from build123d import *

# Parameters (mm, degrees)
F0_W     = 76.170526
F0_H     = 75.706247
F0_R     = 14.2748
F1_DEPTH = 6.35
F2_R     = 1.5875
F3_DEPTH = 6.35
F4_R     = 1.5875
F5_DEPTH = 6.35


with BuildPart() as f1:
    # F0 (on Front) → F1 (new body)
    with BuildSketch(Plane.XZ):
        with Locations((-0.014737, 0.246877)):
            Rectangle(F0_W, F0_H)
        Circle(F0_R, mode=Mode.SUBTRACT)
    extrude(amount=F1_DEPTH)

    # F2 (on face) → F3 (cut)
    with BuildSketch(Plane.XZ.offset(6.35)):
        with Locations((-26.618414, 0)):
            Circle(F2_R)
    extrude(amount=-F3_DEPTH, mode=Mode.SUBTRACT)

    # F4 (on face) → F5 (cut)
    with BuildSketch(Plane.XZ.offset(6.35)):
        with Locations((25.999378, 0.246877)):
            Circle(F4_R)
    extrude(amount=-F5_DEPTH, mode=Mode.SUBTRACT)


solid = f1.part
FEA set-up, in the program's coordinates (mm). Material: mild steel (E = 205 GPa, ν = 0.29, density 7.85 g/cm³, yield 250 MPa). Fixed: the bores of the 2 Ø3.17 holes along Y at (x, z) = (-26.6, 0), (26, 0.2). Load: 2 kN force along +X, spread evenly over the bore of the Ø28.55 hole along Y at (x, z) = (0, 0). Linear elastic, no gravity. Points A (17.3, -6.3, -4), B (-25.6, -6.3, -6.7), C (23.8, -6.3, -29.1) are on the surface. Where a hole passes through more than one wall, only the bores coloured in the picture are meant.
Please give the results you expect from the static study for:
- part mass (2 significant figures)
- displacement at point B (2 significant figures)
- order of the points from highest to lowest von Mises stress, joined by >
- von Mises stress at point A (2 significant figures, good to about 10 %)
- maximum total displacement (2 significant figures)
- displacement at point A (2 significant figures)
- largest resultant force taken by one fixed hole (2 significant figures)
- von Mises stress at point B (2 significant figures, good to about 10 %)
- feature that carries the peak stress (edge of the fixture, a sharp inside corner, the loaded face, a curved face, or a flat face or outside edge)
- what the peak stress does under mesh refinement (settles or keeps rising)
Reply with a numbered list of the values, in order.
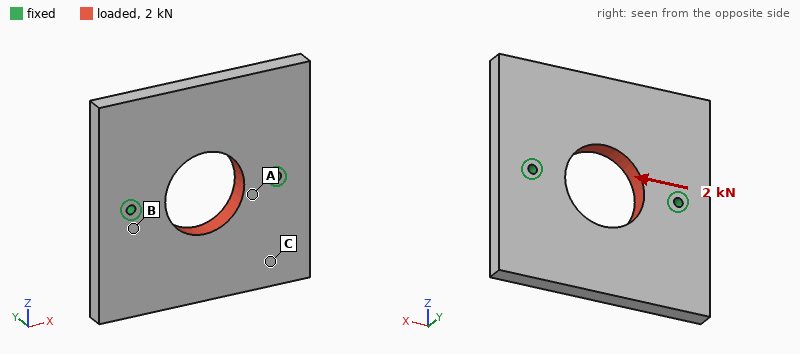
1. 250 g
2. 0.42 µm
3. A > B > C
4. 7.5 MPa
5. 1.1 µm
6. 0.47 µm
7. 1.0 kN
8. 4.5 MPa
9. edge of the fixture
10. keeps rising
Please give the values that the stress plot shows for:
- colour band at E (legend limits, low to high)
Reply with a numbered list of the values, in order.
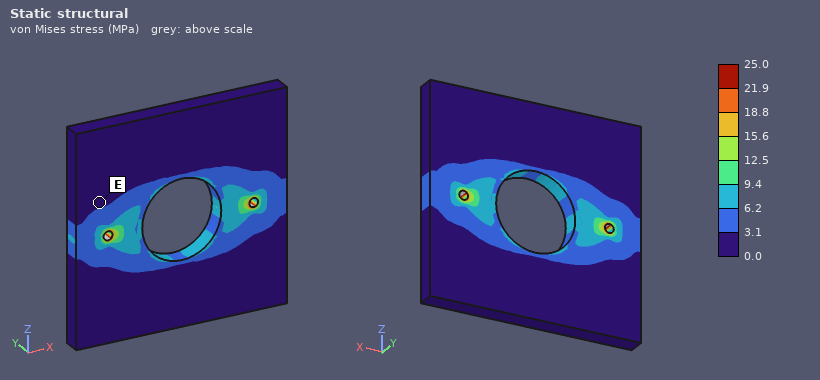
1. 0.0 to 3.1 MPa
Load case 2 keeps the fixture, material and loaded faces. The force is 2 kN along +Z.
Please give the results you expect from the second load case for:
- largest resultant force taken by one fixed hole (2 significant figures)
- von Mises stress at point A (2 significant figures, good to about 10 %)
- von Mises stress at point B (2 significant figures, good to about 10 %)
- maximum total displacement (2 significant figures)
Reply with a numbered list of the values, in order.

1. 1.0 kN
2. 6.8 MPa
3. 7.4 MPa
4. 1.1 µm
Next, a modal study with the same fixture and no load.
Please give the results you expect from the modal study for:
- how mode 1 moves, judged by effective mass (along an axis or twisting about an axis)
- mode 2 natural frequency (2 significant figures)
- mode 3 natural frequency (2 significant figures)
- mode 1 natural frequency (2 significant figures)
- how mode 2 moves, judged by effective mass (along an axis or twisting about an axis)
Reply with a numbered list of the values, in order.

1. twisting about X
2. 3000 Hz
3. 4500 Hz
4. 2300 Hz
5. along Y
